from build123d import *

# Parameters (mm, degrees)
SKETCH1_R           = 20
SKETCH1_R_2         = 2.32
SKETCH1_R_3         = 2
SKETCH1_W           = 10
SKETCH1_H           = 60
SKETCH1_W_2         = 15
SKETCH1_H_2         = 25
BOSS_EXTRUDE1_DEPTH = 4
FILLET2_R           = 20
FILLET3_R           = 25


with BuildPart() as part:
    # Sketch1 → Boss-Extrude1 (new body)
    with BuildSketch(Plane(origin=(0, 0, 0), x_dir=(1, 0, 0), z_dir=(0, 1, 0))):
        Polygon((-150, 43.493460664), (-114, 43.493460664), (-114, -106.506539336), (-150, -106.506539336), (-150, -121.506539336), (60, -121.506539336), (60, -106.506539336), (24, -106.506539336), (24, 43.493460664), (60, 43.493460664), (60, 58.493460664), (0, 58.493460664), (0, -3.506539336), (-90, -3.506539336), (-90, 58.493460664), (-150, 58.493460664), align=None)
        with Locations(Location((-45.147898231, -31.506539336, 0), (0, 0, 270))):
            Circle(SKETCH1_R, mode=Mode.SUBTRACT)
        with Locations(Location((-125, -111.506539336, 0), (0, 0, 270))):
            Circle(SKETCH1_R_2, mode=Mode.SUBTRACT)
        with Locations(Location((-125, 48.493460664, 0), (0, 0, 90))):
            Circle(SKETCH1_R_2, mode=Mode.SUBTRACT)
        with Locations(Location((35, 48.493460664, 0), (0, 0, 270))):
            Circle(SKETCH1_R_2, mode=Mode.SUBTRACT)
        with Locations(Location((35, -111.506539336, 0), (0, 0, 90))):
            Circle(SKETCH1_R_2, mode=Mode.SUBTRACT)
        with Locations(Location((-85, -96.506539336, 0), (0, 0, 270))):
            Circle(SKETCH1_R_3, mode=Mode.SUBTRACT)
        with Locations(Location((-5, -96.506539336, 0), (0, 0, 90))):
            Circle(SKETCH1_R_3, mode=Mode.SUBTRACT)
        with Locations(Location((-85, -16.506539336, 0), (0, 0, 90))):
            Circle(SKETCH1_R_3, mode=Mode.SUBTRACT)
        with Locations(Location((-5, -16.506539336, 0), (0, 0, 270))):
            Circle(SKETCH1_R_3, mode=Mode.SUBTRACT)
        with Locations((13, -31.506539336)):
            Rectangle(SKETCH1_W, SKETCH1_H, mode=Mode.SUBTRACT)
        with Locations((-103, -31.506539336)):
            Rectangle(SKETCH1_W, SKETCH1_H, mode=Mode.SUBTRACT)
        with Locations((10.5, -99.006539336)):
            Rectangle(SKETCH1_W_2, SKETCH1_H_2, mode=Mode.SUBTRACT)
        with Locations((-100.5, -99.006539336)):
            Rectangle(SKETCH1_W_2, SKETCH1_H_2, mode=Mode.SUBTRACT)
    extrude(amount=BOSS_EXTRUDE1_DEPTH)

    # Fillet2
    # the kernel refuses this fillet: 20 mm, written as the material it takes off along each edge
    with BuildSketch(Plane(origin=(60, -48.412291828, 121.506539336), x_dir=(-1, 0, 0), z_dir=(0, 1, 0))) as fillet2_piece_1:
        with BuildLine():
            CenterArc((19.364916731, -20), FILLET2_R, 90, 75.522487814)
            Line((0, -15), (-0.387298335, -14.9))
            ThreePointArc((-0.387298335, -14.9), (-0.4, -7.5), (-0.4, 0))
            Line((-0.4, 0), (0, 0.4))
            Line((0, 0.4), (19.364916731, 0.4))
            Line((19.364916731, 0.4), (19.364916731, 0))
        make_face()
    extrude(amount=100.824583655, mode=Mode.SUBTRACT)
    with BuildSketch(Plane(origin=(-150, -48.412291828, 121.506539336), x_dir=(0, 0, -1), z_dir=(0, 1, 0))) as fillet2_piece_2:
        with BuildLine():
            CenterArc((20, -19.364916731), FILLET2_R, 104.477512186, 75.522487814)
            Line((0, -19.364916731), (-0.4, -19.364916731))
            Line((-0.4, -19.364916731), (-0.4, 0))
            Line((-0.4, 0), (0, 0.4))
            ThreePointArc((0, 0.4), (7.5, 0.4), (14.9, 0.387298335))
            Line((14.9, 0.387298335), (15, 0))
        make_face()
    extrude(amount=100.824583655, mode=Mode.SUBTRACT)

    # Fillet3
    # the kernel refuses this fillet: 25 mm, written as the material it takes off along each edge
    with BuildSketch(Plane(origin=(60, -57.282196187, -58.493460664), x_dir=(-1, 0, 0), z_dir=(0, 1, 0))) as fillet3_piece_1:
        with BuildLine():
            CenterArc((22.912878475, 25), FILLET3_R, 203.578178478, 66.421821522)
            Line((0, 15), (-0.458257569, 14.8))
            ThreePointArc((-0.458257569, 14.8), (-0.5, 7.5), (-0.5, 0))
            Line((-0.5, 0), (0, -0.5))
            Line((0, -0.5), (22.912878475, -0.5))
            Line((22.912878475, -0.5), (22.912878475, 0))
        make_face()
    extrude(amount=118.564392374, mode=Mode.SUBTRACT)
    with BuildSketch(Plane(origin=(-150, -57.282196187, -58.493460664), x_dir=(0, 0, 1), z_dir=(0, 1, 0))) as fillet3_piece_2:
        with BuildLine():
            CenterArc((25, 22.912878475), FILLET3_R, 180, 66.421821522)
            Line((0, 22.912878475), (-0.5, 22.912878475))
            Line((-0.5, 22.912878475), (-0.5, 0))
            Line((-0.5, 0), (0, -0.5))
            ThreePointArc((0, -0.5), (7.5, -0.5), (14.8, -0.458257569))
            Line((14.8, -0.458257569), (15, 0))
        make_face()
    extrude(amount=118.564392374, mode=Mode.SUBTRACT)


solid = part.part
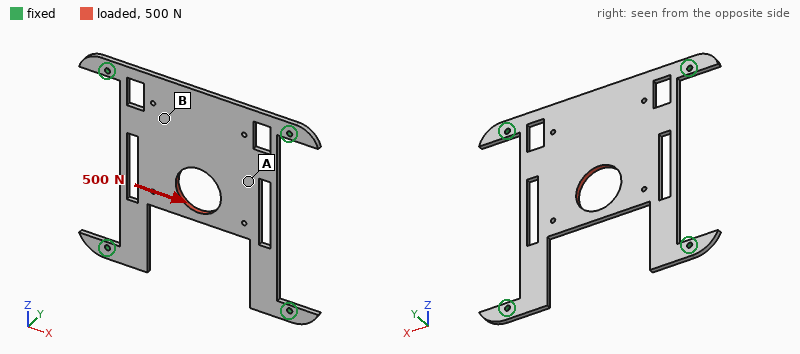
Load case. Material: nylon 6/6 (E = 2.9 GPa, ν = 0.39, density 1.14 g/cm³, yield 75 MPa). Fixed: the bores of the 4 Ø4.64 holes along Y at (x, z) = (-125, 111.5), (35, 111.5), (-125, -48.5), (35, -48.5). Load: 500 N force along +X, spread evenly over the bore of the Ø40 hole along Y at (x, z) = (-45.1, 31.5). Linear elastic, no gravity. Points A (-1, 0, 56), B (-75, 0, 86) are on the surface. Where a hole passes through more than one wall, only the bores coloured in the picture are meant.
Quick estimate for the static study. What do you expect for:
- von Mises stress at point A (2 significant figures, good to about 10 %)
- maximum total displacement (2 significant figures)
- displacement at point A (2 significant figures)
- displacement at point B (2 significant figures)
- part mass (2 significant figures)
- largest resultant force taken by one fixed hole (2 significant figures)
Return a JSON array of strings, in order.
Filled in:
["2.9 MPa", "0.56 mm", "0.34 mm", "0.23 mm", "81 g", "230 N"]
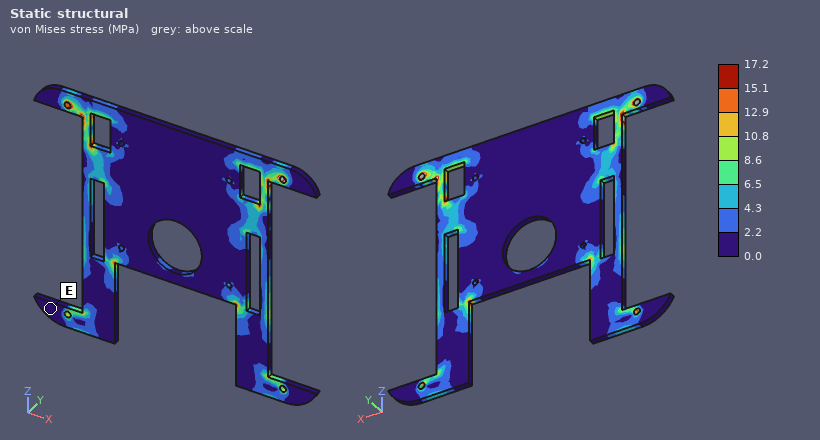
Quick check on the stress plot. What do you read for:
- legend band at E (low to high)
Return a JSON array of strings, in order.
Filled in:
["0.0 to 2.2 MPa"]
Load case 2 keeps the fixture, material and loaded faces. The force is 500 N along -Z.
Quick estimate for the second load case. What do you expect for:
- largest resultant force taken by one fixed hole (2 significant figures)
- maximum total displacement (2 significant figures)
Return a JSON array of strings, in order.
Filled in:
["150 N", "0.23 mm"]
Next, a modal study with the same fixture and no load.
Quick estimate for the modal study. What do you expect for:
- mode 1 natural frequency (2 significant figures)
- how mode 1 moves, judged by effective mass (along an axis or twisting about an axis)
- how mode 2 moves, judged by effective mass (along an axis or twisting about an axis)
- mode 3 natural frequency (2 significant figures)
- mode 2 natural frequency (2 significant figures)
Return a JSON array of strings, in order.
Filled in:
["120 Hz", "along Y", "twisting about Z", "260 Hz", "230 Hz"]
